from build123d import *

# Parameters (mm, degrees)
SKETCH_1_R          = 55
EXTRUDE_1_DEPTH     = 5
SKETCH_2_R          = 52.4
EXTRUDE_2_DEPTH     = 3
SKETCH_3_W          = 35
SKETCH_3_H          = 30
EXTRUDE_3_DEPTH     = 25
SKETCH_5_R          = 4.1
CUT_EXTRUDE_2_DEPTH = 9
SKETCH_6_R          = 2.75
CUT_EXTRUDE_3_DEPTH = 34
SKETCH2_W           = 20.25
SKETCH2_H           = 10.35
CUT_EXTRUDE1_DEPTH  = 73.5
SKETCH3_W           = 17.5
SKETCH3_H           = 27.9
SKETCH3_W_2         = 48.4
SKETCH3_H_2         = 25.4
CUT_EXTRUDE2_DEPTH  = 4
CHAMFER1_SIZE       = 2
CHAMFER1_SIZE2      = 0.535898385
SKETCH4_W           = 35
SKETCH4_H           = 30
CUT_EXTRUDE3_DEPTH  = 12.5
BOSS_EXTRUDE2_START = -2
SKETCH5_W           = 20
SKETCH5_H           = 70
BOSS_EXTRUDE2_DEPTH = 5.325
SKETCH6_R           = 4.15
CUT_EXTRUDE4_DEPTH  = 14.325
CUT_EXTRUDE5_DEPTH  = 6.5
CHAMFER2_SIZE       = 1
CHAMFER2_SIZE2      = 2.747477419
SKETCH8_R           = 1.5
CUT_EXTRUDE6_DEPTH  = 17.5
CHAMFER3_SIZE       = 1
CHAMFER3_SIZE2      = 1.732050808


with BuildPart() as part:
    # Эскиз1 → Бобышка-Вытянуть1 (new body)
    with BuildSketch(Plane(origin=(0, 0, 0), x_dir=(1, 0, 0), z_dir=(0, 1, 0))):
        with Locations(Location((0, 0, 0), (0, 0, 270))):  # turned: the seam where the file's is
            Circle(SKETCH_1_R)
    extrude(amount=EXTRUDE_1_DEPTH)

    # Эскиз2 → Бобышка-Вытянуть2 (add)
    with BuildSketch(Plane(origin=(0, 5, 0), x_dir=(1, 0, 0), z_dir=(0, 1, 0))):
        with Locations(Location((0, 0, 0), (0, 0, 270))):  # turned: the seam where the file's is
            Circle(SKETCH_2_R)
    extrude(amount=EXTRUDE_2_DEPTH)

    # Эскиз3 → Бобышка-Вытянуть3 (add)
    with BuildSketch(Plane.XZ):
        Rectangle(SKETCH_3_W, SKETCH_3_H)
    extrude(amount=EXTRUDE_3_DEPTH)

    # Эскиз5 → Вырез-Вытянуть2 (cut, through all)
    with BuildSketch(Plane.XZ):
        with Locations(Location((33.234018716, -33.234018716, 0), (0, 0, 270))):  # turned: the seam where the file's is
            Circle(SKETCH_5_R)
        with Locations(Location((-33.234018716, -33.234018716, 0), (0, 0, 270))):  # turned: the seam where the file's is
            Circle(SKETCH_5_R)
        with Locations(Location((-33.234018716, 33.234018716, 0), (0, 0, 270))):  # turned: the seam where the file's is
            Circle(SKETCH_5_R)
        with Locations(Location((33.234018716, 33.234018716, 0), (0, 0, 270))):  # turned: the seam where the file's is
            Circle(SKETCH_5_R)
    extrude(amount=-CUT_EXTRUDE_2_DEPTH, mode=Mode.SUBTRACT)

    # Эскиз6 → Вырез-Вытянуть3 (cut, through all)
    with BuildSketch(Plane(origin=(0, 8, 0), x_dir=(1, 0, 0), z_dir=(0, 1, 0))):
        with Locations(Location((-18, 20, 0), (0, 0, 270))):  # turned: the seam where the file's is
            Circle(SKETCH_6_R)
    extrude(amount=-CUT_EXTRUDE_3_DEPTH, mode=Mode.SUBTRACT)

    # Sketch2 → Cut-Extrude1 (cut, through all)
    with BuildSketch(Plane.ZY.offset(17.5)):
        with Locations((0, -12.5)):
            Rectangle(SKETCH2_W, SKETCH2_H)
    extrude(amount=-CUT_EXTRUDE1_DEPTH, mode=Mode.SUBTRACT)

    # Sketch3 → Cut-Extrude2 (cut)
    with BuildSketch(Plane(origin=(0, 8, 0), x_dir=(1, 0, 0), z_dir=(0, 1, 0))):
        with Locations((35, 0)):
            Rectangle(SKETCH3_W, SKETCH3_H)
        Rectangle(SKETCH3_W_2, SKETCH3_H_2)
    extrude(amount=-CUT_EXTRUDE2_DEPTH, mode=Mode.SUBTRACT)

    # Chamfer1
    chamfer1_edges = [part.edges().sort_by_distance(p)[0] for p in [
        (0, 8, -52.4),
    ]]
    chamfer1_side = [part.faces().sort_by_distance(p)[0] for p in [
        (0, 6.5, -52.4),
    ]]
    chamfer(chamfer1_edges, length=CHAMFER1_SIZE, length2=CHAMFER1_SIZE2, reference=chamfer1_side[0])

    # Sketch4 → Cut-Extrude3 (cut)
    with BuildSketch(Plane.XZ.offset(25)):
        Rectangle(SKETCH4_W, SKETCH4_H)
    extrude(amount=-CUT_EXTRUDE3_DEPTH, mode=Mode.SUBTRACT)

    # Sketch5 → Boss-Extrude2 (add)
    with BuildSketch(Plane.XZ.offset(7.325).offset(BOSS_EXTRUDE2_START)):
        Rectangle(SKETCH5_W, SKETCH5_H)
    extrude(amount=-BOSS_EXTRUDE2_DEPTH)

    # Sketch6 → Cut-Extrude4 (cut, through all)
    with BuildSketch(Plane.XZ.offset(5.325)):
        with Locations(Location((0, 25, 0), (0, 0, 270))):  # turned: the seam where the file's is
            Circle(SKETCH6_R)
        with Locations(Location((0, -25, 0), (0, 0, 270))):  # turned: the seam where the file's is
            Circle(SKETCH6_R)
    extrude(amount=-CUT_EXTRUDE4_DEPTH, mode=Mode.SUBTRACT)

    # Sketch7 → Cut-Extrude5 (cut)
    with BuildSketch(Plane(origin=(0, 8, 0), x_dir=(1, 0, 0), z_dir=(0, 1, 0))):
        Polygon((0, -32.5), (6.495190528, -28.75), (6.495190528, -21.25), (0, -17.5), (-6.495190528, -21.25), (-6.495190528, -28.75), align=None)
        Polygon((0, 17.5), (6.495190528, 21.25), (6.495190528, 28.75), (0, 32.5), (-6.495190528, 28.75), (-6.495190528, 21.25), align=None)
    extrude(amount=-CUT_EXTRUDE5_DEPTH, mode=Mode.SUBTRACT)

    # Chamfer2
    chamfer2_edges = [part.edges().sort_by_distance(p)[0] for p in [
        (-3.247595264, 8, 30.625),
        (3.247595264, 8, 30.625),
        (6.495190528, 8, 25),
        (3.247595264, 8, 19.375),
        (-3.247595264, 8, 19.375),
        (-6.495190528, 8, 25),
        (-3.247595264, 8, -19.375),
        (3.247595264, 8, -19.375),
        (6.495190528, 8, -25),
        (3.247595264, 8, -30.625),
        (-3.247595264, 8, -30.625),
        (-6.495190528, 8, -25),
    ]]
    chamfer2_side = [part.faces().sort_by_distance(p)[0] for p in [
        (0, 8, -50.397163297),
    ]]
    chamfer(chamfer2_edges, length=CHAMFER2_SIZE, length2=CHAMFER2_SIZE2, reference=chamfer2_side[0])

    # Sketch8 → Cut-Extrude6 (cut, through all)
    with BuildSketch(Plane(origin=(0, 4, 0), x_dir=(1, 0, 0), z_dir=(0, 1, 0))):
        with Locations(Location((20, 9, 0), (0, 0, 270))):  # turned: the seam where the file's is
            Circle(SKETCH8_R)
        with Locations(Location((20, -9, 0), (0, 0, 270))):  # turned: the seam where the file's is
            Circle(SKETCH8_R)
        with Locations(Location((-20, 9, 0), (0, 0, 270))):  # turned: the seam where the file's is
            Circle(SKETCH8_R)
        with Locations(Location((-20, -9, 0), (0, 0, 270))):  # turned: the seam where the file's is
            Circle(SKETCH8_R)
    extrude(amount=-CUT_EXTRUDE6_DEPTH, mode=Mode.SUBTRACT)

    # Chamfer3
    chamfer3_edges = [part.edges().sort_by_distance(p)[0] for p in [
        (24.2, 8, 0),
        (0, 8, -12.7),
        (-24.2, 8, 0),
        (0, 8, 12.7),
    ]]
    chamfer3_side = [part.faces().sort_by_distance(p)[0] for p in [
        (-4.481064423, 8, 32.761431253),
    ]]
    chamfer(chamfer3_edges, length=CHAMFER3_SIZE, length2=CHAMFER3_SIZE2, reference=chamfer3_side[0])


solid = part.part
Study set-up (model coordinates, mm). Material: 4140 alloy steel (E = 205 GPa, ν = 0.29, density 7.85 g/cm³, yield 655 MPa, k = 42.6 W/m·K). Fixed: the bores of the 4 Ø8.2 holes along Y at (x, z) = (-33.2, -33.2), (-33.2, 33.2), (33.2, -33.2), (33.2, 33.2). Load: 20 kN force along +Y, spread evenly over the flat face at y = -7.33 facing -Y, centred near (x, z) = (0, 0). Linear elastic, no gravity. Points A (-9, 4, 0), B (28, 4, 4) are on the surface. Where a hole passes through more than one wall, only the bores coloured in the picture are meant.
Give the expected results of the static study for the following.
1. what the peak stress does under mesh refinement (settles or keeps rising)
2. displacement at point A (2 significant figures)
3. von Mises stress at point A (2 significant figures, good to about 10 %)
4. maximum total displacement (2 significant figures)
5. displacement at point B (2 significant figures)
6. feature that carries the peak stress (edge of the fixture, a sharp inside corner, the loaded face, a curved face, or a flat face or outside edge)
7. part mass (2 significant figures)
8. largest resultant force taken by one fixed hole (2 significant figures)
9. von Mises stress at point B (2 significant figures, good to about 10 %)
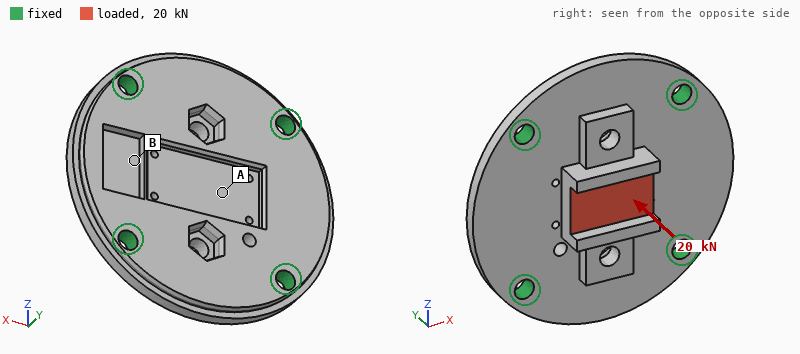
keeps rising
64 µm
91 MPa
66 µm
40 µm
edge of the fixture
590 g
8.0 kN
45 MPa
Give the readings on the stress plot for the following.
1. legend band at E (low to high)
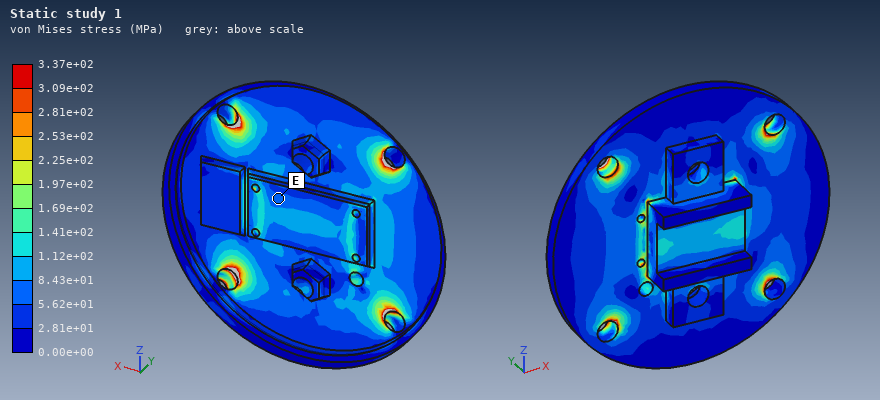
5.62e+01 to 8.43e+01 MPa
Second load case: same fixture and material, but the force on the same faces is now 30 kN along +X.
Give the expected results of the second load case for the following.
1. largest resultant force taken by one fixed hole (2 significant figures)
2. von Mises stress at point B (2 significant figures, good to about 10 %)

9.2 kN
34 MPa
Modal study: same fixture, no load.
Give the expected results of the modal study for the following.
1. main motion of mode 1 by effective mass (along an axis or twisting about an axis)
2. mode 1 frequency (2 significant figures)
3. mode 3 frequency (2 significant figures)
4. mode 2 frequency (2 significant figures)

along Y
6600 Hz
8200 Hz
8200 Hz
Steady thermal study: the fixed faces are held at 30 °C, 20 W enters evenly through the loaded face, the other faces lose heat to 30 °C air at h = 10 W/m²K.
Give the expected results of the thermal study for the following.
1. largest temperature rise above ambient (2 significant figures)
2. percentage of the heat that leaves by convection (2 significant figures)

21 K
8.0 %
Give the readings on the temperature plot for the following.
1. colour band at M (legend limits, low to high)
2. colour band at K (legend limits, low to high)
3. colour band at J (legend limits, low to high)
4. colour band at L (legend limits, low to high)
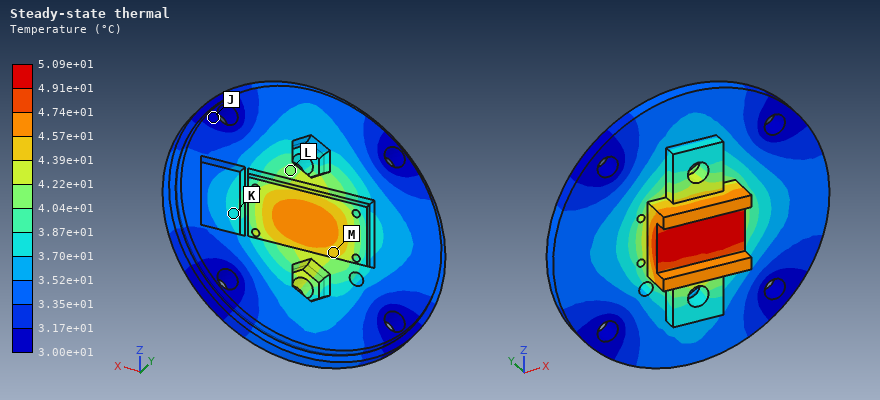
4.39e+01 to 4.57e+01 °C
3.70e+01 to 3.87e+01 °C
3.00e+01 to 3.17e+01 °C
4.04e+01 to 4.22e+01 °C
